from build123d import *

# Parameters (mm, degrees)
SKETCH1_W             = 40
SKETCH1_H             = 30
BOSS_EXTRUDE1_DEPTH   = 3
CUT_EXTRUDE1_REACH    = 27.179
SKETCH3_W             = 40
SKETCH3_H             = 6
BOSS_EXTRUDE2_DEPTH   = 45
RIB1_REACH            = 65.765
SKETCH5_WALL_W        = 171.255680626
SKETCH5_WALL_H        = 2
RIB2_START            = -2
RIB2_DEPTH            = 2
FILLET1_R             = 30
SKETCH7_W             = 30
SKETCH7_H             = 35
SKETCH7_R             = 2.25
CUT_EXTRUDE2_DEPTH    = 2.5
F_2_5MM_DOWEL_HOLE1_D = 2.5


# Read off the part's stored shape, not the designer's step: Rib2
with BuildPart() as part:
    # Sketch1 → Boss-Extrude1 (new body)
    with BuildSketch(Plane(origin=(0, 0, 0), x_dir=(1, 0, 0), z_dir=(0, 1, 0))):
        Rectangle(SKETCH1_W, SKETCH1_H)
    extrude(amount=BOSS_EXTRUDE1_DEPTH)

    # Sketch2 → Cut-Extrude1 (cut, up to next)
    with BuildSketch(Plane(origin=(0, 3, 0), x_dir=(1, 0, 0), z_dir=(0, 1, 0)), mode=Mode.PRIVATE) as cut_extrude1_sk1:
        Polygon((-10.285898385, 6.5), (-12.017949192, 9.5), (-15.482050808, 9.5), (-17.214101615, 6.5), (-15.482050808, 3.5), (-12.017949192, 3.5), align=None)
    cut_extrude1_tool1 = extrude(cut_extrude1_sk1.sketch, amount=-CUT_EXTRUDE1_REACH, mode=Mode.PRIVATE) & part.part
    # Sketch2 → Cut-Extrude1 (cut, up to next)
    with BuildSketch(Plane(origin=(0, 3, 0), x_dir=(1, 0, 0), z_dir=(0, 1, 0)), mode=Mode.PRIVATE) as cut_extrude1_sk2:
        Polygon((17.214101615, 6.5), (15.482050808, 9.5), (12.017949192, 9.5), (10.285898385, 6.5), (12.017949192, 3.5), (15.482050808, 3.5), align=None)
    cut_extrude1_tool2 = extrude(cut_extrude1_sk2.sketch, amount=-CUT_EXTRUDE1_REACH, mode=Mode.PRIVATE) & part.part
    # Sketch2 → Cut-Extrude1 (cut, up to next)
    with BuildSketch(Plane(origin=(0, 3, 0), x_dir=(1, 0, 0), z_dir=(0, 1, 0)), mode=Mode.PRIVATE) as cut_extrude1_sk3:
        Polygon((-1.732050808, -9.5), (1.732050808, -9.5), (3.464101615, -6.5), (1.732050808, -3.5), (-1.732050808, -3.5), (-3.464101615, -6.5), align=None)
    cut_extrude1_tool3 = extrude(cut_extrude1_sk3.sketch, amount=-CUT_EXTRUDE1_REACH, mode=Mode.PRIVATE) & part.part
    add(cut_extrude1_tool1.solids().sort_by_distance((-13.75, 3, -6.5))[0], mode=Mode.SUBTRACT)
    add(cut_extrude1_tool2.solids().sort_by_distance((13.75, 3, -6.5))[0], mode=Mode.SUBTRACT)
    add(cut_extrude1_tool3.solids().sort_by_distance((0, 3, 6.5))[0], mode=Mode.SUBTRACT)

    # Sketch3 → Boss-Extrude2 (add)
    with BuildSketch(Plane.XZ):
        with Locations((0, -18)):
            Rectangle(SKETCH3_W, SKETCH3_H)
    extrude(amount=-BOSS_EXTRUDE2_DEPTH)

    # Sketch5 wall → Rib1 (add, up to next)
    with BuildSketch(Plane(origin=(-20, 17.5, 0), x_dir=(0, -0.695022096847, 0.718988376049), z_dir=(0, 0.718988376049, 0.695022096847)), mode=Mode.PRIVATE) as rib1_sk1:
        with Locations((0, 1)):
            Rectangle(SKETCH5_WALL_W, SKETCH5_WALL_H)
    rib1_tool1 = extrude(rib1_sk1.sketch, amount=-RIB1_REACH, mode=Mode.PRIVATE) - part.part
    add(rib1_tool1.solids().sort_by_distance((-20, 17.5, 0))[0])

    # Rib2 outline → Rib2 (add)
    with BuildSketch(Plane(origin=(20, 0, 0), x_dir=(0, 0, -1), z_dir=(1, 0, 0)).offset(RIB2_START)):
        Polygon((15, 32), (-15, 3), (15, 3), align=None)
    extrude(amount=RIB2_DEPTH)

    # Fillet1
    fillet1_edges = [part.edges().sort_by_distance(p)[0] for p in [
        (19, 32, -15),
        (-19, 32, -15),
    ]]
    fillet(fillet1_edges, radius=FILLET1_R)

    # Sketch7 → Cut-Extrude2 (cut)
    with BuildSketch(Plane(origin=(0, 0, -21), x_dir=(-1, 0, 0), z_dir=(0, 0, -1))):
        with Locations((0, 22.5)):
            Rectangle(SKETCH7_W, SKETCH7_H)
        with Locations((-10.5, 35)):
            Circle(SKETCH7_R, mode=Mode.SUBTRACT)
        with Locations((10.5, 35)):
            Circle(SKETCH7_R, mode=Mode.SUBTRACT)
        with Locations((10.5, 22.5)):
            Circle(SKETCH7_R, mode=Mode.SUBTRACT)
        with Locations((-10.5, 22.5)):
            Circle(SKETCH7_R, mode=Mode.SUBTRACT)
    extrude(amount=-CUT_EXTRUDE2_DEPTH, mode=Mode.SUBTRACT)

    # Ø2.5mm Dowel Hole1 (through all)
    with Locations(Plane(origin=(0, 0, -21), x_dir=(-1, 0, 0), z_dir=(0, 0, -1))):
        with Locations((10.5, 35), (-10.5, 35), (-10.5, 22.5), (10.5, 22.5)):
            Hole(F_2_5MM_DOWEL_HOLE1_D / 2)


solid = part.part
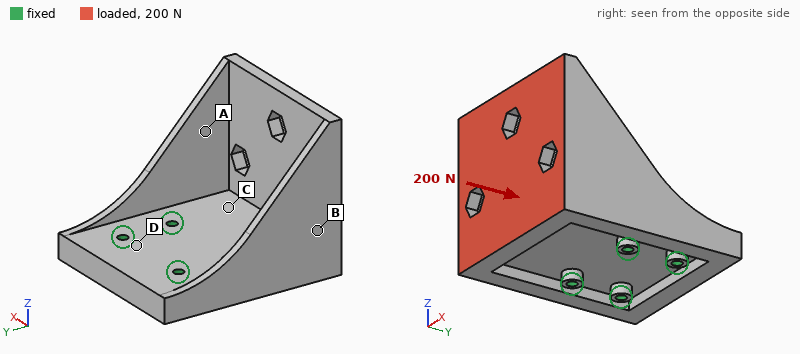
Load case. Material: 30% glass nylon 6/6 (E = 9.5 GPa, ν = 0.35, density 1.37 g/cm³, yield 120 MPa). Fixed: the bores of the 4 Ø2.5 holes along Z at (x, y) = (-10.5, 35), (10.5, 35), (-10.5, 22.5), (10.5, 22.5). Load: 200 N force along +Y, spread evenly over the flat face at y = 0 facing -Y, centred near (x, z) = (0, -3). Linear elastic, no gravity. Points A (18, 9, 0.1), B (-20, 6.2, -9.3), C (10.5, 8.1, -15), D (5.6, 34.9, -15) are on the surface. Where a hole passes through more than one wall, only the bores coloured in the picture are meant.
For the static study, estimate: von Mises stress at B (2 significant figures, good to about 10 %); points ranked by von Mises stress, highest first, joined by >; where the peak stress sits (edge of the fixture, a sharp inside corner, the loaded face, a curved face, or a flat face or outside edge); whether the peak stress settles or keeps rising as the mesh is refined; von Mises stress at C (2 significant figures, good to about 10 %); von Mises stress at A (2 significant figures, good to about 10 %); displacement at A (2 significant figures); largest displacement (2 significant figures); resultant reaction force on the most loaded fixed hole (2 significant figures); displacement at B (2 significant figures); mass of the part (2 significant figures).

4.4 MPa
A > B > C > D
edge of the fixture
keeps rising
3.0 MPa
6.9 MPa
0.096 mm
0.28 mm
100 N
0.071 mm
18 g
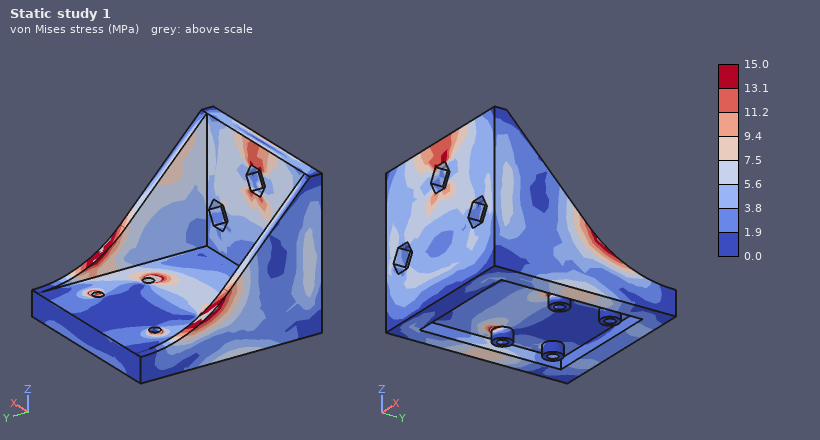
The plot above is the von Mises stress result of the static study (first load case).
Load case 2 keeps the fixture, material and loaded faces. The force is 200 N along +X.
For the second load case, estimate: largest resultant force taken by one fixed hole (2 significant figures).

210 N
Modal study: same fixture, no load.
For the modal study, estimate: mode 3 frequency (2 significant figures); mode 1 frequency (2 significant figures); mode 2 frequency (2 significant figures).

3700 Hz
1700 Hz
1700 Hz
